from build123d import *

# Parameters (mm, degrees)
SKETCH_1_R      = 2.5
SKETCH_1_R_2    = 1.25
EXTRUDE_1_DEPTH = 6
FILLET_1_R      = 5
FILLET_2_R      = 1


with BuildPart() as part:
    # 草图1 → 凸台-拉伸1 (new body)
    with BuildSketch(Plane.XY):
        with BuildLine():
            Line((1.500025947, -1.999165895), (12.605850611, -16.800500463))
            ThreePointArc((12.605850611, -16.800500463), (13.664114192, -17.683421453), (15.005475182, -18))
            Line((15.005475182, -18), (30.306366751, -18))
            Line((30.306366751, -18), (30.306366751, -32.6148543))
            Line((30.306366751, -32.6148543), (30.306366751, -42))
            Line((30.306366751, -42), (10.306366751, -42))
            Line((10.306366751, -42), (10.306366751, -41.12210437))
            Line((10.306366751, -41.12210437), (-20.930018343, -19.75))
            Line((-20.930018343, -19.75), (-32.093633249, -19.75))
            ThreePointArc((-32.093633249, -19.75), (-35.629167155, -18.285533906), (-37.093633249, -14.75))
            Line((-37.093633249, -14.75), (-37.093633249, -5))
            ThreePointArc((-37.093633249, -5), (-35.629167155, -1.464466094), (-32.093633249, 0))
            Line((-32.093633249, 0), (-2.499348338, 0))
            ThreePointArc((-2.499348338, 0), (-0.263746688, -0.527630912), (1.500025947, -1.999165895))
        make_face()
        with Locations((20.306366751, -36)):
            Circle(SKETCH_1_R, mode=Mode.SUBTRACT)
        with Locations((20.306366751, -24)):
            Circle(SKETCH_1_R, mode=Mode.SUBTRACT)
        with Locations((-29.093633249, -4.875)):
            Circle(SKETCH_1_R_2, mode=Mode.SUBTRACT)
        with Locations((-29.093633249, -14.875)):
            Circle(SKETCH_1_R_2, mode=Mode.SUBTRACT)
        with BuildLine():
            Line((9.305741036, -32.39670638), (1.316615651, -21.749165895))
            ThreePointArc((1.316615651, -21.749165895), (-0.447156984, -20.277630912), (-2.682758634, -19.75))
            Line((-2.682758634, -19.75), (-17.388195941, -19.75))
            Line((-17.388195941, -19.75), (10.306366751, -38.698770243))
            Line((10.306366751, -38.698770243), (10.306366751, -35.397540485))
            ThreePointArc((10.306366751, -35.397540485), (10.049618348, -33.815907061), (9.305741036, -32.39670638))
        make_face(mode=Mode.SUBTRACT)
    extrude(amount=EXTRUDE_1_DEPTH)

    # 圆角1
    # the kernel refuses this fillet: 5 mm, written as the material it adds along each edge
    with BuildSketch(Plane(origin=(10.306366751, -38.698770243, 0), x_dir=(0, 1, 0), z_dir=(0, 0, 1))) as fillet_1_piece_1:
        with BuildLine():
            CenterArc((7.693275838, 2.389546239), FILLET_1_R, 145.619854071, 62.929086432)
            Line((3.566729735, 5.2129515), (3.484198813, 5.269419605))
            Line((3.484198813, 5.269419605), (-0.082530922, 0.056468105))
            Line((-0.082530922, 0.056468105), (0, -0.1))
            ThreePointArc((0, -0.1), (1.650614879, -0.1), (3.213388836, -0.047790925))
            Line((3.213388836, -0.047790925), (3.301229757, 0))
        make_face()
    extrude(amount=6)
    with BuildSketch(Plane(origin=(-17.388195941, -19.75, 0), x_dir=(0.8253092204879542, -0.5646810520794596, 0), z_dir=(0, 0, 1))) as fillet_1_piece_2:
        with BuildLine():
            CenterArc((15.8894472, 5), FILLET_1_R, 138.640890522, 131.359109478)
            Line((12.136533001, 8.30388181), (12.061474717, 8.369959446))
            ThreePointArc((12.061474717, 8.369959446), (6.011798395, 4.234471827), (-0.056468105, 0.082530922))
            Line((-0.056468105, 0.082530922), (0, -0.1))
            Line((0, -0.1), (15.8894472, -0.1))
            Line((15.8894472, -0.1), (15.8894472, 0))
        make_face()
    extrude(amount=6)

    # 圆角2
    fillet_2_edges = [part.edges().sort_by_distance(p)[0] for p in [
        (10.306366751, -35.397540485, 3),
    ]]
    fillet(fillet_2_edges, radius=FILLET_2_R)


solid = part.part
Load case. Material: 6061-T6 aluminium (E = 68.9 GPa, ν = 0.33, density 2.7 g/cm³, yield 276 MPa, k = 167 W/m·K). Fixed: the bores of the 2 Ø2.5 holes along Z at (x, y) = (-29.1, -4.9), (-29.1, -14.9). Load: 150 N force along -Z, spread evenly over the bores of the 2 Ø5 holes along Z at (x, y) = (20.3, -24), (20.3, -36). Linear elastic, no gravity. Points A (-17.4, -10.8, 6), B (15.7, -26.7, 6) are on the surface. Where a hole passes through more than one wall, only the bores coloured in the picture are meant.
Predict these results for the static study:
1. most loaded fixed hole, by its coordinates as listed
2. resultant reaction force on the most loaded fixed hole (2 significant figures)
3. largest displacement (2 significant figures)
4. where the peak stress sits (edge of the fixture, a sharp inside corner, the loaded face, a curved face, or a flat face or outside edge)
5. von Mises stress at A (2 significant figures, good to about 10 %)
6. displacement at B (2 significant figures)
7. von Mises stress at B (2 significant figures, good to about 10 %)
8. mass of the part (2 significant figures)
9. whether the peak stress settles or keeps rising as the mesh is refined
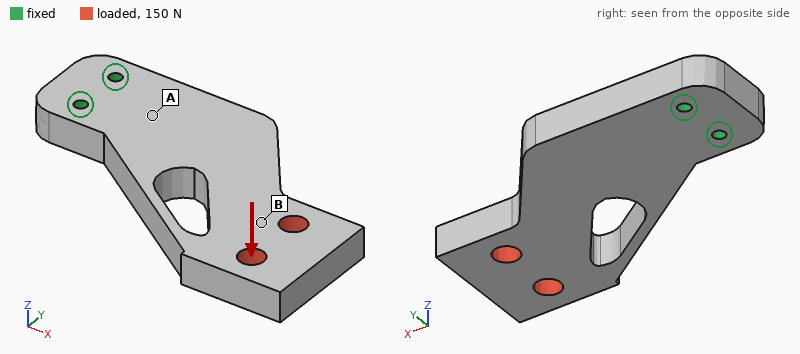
(-29.1, -14.9)
270 N
0.43 mm
edge of the fixture
47 MPa
0.26 mm
10 MPa
24 g
keeps rising
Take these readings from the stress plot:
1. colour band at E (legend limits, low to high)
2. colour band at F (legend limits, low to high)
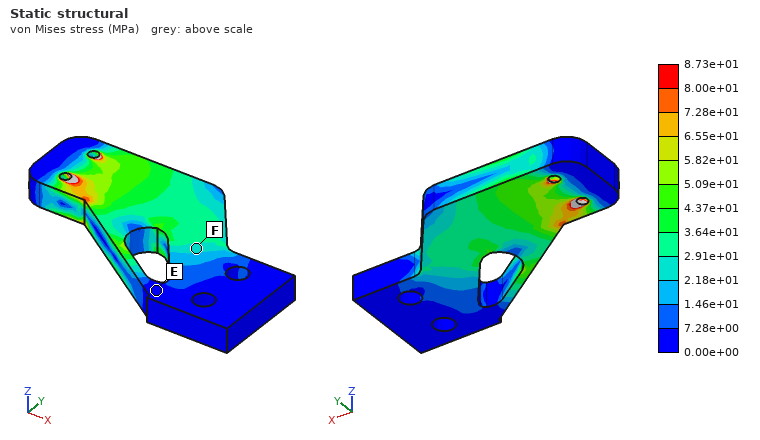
0.00e+00 to 7.28e+00 MPa
2.18e+01 to 2.91e+01 MPa
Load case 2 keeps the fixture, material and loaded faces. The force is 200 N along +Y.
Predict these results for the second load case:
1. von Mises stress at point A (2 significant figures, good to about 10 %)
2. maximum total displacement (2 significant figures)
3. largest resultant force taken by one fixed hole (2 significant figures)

7.2 MPa
55 µm
870 N
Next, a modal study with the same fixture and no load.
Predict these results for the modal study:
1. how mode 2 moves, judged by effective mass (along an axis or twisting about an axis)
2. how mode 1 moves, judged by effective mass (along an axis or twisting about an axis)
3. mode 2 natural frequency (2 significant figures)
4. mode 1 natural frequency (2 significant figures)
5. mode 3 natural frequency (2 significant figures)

along Y
along Z
3400 Hz
1200 Hz
4800 Hz
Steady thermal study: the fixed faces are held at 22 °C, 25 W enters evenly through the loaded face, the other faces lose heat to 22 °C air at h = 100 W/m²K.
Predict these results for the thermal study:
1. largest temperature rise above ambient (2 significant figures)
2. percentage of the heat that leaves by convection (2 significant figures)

51 K
42 %
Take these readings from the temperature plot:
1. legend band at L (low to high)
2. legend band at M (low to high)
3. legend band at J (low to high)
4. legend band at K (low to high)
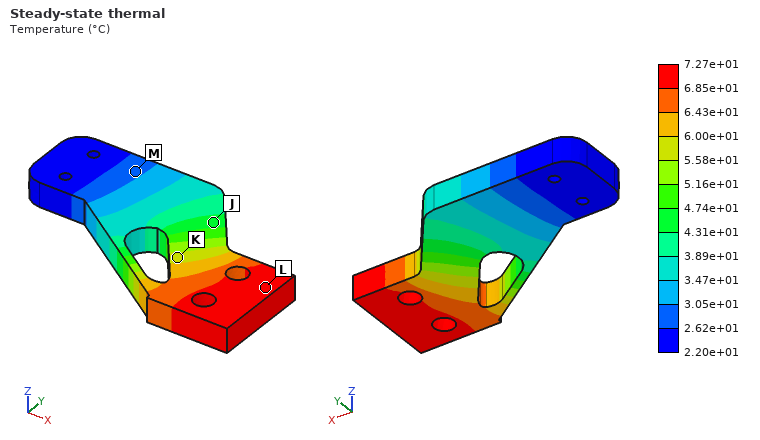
6.85e+01 to 7.27e+01 °C
2.62e+01 to 3.05e+01 °C
4.31e+01 to 4.74e+01 °C
5.58e+01 to 6.00e+01 °C
